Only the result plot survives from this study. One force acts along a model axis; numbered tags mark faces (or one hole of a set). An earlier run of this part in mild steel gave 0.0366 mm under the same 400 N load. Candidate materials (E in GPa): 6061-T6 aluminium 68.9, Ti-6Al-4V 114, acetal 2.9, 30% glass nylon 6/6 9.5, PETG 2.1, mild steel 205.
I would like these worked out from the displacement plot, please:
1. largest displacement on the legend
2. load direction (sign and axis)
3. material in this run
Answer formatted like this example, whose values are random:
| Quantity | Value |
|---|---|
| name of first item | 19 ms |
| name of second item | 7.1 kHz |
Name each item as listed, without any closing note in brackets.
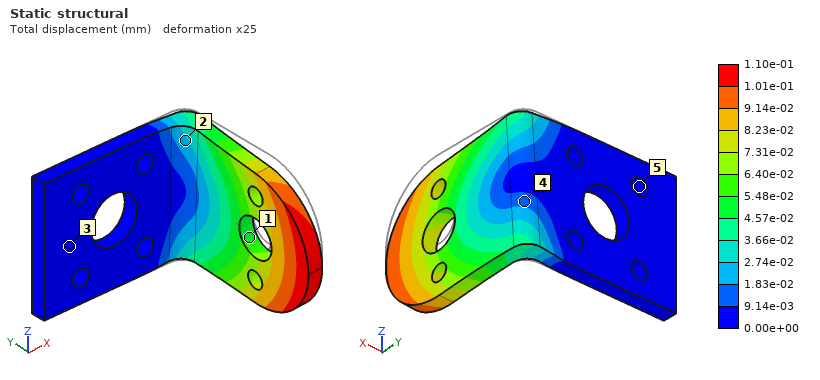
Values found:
| Quantity | Value |
|---|---|
| largest displacement on the legend | 1.10e-01 mm |
| load direction | -Z |
| material in this run | 6061-T6 aluminium |
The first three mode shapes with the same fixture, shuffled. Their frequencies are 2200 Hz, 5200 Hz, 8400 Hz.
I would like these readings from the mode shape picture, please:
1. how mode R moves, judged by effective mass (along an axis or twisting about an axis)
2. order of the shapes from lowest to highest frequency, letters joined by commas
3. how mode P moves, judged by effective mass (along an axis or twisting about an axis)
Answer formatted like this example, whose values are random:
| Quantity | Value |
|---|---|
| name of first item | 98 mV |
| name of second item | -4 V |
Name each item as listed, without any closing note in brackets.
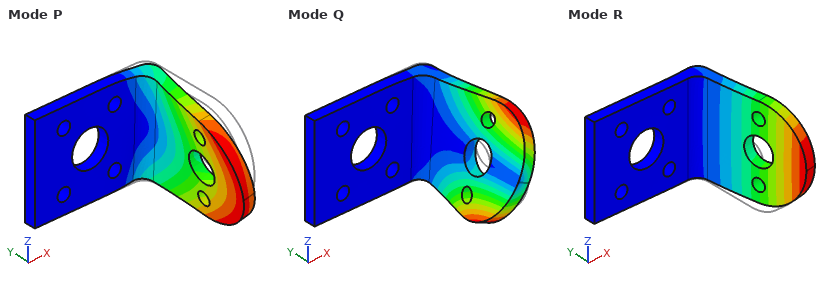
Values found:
| Quantity | Value |
|---|---|
| how mode R moves, judged by effective mass | along X |
| order of the shapes from lowest to highest frequency, letters joined by commas | R, P, Q |
| how mode P moves, judged by effective mass | along Z |
